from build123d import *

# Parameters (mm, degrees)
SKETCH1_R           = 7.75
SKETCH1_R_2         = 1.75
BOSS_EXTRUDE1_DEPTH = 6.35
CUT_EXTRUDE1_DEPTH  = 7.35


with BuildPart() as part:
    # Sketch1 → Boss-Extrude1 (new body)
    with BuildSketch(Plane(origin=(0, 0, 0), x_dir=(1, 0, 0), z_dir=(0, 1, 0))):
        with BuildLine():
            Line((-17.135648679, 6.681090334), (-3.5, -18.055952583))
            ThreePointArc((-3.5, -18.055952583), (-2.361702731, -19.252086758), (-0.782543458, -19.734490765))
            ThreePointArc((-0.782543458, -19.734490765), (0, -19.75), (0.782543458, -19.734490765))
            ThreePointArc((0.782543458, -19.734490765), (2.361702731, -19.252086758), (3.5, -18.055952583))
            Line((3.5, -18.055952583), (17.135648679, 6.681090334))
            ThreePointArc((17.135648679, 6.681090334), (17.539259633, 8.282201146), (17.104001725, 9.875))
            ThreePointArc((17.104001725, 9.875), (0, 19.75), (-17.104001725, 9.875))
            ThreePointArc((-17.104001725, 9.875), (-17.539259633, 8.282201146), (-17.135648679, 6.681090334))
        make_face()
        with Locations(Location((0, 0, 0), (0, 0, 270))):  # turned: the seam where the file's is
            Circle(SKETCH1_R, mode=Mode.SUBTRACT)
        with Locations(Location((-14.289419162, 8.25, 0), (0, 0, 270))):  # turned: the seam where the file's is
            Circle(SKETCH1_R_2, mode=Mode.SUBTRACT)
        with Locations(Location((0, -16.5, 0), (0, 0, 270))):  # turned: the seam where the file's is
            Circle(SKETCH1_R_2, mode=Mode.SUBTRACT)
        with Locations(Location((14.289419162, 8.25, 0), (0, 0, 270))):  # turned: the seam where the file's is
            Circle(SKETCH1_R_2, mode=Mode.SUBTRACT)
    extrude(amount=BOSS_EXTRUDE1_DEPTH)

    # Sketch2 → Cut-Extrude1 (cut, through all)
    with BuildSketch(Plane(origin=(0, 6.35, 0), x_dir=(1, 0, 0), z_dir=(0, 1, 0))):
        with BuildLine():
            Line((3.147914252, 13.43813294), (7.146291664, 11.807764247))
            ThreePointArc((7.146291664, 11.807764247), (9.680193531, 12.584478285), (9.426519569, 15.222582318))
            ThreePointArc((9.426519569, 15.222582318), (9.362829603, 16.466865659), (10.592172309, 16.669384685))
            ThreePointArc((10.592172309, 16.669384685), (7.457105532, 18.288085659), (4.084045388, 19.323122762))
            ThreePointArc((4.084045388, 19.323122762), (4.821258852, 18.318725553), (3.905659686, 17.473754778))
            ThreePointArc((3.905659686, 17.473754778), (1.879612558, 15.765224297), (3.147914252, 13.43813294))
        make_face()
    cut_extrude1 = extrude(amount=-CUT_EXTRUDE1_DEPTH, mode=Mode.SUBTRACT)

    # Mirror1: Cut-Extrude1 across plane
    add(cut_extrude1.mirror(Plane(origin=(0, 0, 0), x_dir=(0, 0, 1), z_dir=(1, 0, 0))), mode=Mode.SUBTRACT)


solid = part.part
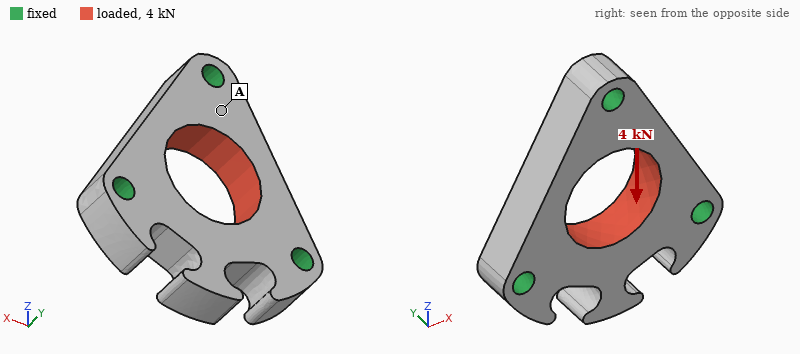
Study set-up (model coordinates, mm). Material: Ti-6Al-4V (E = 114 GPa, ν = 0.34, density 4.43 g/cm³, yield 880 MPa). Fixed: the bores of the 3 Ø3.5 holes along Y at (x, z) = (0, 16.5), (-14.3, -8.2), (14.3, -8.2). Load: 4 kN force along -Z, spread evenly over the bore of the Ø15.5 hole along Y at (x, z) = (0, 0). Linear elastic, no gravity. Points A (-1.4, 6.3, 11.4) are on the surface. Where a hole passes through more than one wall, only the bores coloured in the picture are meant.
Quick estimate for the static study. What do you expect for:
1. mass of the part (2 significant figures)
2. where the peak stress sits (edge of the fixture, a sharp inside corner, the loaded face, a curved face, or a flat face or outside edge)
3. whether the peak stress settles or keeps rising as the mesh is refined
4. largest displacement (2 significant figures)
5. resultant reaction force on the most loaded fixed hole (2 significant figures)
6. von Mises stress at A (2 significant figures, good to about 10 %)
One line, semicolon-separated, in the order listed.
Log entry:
16 g; edge of the fixture; keeps rising; 9.0 µm; 1.4 kN; 17 MPa
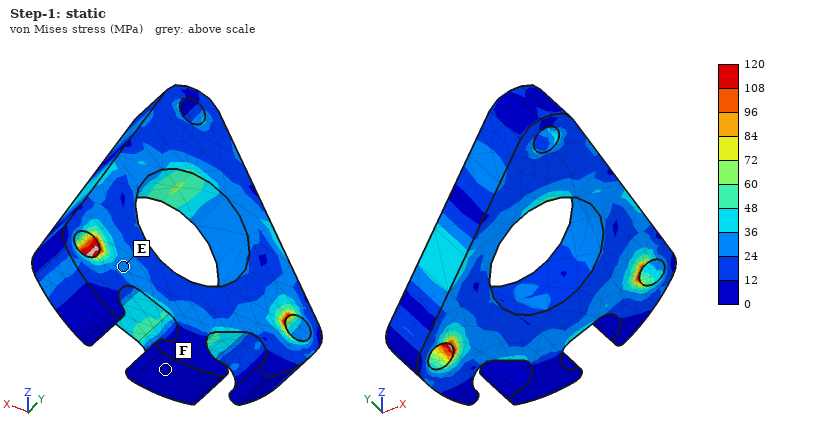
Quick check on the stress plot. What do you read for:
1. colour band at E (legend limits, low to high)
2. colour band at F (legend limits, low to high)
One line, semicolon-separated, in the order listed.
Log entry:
24 to 36 MPa; 0 to 12 MPa
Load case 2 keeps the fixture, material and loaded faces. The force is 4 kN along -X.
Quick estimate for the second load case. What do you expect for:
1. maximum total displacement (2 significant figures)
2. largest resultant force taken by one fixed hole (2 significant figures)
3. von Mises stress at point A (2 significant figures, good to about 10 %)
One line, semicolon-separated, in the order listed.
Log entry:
10 µm; 1.4 kN; 33 MPa
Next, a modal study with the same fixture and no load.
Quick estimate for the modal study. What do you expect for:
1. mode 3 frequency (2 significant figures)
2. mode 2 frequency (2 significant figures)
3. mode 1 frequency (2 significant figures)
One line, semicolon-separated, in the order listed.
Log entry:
33 kHz; 32 kHz; 19 kHz
